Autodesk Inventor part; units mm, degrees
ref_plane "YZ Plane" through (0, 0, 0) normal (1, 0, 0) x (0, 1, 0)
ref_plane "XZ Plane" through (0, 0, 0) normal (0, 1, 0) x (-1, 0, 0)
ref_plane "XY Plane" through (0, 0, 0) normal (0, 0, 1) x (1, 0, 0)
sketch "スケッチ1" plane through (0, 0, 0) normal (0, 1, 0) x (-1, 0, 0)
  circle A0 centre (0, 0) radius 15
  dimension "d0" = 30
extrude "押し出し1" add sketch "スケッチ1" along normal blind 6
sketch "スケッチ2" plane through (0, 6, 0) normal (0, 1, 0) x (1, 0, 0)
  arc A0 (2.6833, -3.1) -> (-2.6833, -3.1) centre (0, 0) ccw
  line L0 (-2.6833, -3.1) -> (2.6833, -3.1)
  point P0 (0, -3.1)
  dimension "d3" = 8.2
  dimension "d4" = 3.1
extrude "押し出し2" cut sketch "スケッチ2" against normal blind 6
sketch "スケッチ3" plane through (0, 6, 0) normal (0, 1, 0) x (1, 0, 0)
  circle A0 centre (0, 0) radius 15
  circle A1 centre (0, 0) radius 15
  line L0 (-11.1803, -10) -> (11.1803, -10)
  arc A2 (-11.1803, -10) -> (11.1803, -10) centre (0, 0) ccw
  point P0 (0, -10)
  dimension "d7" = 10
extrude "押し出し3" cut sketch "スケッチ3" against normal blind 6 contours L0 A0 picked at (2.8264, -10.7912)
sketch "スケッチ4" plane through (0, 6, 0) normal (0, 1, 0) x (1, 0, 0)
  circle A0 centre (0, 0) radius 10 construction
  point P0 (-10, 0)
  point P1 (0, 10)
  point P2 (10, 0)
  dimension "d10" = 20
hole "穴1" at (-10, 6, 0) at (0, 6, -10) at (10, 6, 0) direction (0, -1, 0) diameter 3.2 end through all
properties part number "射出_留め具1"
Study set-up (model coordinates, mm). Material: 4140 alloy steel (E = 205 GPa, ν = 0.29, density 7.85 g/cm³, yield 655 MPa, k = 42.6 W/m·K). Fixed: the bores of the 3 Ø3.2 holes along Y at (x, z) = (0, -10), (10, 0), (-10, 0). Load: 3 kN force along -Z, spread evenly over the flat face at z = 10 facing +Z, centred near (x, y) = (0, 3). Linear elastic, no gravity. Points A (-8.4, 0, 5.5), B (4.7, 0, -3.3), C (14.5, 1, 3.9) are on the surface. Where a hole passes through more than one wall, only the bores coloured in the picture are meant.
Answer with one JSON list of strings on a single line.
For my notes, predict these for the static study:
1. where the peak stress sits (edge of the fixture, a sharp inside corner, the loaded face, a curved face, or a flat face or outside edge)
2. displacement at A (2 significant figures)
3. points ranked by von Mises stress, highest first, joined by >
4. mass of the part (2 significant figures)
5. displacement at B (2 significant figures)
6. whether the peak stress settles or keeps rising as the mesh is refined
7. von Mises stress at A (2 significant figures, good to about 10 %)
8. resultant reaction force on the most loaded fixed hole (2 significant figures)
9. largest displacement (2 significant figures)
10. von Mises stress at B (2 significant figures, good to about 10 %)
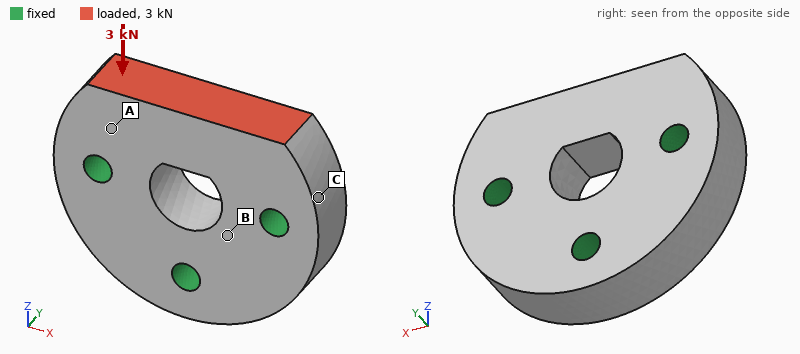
["edge of the fixture", "0.72 µm", "A > B > C", "26 g", "0.36 µm", "keeps rising", "28 MPa", "1.4 kN", "2.2 µm", "13 MPa"]
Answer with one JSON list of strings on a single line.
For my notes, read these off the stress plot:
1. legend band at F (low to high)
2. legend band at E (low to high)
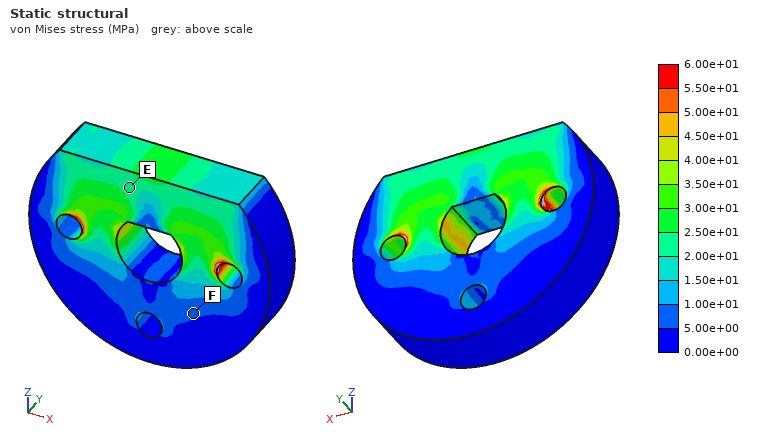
["5.00e+00 to 1.00e+01 MPa", "2.00e+01 to 2.50e+01 MPa"]
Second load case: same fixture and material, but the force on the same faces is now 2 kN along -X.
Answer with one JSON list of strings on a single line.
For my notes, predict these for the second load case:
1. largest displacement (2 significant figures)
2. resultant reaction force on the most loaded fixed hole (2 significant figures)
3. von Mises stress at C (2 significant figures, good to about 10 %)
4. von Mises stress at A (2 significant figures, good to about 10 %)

["2.7 µm", "1.3 kN", "18 MPa", "20 MPa"]
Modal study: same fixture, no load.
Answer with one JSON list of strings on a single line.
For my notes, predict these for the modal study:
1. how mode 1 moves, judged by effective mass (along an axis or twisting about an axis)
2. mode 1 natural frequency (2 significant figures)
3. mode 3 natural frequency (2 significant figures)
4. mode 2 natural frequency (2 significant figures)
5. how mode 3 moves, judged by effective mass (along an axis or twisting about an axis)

["along Y", "34 kHz", "61 kHz", "54 kHz", "along X"]
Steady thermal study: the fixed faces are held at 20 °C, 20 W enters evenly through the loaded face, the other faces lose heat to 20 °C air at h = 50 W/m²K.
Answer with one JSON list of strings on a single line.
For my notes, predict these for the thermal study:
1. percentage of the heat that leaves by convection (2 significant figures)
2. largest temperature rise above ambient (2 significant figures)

["3.5 %", "41 K"]
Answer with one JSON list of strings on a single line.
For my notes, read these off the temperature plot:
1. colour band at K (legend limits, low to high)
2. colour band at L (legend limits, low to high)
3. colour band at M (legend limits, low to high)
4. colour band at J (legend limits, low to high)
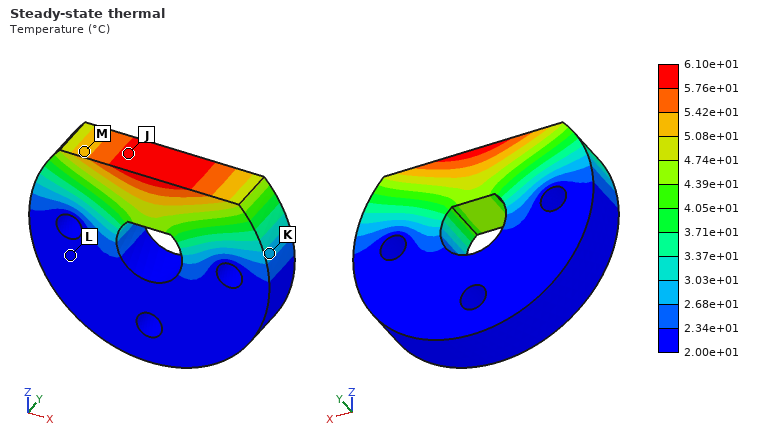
["2.68e+01 to 3.03e+01 °C", "2.00e+01 to 2.34e+01 °C", "5.08e+01 to 5.42e+01 °C", "5.76e+01 to 6.10e+01 °C"]
